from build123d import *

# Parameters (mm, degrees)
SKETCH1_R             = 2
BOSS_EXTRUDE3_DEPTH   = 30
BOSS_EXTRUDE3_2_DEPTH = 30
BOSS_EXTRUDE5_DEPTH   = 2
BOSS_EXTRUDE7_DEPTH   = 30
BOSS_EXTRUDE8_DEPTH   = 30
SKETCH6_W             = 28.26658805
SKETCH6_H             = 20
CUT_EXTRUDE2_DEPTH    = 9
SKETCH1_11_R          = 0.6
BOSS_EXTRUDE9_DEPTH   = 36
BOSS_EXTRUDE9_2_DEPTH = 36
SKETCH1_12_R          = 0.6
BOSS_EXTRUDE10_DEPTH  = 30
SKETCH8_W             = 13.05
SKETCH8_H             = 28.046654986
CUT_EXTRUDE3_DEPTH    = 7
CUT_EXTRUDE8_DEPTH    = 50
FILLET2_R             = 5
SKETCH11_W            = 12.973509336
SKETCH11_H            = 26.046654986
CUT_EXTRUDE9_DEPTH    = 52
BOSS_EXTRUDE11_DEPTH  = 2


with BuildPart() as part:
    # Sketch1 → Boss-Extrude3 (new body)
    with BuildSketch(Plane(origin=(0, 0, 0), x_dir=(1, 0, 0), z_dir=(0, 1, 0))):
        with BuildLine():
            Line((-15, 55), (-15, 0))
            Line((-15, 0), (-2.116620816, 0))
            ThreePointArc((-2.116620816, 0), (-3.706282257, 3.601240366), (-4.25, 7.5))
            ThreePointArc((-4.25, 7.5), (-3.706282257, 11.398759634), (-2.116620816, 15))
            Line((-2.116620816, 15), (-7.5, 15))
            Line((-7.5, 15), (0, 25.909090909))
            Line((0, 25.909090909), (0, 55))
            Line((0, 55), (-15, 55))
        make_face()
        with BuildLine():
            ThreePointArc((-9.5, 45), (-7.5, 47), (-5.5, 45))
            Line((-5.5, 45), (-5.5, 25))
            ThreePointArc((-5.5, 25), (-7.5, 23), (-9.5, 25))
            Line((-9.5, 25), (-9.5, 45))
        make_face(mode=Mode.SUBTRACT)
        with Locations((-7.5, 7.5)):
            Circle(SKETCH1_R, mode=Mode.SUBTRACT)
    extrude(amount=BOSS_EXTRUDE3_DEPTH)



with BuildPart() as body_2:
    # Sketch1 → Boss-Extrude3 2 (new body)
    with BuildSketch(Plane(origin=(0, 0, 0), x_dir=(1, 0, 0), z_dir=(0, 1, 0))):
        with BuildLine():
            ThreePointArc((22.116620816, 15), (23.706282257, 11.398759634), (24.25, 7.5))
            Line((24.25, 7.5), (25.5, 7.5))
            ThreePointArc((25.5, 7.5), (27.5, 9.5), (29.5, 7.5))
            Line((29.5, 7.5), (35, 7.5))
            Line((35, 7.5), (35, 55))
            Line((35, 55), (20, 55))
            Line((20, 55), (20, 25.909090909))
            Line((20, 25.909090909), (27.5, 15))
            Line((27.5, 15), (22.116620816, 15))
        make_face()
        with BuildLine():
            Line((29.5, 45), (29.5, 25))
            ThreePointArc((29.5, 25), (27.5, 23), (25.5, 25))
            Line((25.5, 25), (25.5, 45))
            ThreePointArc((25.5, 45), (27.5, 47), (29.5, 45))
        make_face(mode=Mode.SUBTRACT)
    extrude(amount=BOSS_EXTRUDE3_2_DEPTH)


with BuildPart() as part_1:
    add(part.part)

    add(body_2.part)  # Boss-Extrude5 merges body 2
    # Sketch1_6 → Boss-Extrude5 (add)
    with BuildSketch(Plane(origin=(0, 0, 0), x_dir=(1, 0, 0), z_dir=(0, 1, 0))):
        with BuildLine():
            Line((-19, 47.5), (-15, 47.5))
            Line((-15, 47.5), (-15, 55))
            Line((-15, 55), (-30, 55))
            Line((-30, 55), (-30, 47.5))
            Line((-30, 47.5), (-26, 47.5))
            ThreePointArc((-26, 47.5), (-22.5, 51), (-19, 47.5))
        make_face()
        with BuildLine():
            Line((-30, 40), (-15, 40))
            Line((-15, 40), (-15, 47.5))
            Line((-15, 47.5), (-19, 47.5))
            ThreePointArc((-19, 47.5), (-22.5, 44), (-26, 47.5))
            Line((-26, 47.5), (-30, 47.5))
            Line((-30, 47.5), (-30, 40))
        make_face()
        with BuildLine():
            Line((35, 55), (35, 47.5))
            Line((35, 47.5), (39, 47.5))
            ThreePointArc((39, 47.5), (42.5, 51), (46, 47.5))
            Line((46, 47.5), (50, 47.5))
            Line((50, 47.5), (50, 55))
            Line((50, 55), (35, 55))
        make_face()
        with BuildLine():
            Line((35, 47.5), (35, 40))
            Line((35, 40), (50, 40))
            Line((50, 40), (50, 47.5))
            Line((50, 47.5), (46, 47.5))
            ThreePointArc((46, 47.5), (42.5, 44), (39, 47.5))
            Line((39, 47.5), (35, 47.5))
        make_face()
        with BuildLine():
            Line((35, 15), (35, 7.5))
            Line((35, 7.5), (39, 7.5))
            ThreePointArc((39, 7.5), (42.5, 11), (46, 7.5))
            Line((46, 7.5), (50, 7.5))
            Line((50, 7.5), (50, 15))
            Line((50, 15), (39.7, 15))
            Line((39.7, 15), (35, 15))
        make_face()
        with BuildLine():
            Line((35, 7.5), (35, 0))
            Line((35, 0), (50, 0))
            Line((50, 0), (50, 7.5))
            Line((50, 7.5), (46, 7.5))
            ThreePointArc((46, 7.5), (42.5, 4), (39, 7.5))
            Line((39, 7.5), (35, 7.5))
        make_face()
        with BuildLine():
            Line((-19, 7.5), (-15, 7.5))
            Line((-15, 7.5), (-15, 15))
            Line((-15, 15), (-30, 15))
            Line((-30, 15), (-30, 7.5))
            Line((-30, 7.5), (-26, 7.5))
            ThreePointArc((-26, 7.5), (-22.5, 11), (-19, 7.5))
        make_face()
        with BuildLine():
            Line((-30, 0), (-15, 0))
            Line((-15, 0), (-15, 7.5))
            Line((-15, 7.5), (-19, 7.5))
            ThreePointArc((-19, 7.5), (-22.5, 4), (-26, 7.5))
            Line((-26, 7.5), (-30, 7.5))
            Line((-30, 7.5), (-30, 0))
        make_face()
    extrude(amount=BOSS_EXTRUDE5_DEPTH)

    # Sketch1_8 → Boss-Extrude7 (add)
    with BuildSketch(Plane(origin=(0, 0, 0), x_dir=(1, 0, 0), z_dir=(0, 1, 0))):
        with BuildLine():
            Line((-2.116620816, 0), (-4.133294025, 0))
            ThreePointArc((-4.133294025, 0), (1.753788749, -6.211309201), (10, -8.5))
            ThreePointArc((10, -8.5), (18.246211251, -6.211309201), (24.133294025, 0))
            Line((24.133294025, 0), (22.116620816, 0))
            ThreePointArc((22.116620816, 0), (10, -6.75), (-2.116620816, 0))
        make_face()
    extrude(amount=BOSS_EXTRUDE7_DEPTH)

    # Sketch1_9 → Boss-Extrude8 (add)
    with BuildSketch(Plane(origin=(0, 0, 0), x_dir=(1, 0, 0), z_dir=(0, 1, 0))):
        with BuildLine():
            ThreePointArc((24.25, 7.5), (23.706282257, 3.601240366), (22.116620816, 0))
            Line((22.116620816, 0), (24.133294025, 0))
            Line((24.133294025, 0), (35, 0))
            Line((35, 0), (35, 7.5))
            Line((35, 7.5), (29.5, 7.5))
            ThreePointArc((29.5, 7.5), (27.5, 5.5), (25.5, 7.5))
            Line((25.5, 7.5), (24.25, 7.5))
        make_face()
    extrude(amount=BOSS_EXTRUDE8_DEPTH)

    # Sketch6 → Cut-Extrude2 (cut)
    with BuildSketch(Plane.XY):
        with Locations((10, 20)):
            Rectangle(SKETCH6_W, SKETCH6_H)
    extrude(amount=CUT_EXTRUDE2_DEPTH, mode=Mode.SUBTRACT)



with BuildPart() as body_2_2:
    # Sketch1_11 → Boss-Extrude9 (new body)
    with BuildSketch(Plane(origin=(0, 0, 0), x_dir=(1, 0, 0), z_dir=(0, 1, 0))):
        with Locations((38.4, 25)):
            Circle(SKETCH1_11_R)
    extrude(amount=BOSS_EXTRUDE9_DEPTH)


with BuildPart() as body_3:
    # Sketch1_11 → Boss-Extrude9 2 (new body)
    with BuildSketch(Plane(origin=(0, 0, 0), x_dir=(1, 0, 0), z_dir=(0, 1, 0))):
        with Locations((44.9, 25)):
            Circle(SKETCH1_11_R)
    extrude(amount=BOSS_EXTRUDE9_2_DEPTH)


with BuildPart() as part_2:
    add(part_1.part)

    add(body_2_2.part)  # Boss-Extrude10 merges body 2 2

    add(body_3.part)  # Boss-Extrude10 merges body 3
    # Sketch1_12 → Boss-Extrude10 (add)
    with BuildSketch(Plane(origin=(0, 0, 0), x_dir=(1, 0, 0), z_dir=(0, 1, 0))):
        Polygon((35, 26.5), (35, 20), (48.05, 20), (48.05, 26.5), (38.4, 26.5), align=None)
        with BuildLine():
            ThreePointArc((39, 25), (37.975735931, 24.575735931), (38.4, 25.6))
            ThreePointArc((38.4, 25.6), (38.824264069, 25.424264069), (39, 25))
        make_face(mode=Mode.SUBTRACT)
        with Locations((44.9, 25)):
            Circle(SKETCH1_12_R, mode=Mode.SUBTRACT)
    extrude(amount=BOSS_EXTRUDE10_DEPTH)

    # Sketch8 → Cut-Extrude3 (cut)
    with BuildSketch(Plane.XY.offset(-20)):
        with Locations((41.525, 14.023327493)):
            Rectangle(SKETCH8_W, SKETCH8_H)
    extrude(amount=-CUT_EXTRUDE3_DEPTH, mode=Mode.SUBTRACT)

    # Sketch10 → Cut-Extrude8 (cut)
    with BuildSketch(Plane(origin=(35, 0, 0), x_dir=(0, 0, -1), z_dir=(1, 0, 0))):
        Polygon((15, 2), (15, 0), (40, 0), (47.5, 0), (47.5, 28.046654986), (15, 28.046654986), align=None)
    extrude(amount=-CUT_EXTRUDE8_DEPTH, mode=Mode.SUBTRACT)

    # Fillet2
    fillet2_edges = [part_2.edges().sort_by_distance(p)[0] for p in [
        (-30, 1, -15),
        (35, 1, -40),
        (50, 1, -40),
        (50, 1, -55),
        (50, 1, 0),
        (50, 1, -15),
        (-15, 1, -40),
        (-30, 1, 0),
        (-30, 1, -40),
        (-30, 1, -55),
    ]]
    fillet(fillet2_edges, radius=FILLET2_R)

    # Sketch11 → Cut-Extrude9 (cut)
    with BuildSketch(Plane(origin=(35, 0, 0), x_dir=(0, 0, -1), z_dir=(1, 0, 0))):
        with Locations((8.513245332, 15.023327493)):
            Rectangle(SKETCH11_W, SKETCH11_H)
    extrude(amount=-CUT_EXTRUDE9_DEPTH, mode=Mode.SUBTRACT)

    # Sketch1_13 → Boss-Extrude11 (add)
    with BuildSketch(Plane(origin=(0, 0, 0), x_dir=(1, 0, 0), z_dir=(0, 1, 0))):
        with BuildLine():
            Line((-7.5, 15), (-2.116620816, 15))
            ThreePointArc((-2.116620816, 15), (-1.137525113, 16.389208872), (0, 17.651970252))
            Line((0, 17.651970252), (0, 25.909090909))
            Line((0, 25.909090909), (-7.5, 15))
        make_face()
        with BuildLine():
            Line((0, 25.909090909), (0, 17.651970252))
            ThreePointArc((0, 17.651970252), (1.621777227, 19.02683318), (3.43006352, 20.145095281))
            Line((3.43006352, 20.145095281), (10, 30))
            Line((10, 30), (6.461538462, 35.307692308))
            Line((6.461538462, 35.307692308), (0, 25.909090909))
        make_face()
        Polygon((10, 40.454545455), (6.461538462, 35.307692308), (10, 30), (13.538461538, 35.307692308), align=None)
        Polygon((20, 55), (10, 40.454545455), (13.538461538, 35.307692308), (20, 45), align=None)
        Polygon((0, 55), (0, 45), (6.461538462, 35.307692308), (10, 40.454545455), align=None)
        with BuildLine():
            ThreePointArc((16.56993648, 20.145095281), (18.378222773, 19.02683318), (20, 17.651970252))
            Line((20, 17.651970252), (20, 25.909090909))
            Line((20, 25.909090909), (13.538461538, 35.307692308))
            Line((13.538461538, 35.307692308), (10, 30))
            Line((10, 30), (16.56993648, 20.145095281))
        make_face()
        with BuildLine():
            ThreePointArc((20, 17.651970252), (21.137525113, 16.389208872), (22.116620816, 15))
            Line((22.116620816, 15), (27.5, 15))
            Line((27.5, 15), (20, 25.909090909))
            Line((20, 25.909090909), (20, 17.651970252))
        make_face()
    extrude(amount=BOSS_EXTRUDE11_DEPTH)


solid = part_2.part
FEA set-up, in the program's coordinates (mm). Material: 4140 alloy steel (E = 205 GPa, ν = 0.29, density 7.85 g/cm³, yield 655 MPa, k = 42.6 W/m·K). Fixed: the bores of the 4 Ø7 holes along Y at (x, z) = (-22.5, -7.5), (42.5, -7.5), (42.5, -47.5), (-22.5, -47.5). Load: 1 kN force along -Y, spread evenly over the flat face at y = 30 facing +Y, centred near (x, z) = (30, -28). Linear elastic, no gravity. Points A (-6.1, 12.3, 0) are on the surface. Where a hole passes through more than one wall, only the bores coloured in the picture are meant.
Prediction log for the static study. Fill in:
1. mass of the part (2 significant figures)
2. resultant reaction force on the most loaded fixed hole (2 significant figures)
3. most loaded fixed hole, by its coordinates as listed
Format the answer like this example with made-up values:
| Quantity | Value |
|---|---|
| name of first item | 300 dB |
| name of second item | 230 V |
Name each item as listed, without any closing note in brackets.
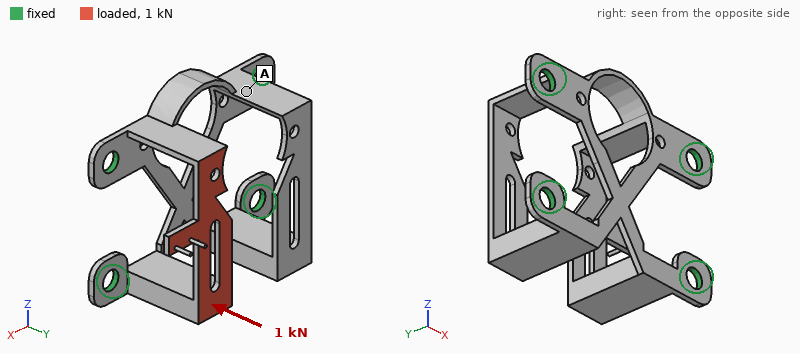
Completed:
| Quantity | Value |
|---|---|
| mass of the part | 110 g |
| resultant reaction force on the most loaded fixed hole | 580 N |
| most loaded fixed hole, by its coordinates as listed | (42.5, -47.5) |
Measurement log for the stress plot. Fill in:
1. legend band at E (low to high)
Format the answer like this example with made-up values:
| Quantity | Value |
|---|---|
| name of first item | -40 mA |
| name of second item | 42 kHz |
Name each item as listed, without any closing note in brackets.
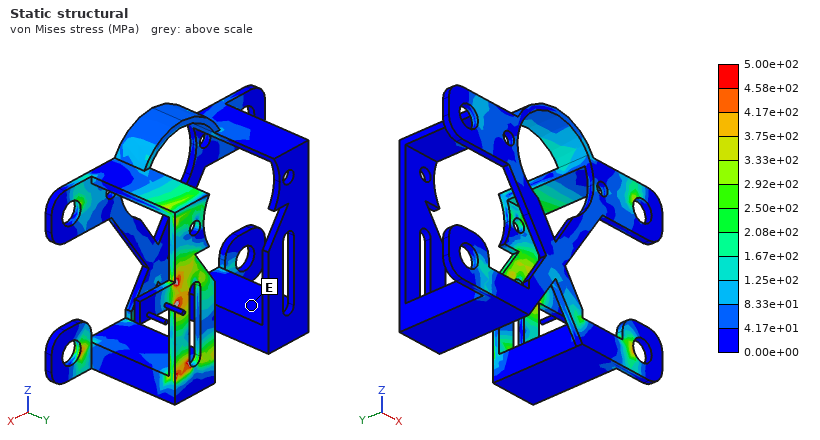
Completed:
| Quantity | Value |
|---|---|
| legend band at E | 0.00e+00 to 4.17e+01 MPa |
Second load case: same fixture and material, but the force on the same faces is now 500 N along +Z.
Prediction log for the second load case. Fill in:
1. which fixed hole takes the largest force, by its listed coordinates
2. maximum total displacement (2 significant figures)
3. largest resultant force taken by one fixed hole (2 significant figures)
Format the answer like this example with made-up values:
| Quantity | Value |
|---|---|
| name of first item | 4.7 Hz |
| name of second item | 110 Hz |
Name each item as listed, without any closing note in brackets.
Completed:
| Quantity | Value |
|---|---|
| which fixed hole takes the largest force, by its listed coordinates | (42.5, -47.5) |
| maximum total displacement | 0.43 mm |
| largest resultant force taken by one fixed hole | 360 N |
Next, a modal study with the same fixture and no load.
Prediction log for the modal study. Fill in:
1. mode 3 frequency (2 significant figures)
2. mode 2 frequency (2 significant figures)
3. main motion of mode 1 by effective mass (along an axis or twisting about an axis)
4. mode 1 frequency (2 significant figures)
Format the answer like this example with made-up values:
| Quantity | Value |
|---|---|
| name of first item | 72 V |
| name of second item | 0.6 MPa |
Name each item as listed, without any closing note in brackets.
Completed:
| Quantity | Value |
|---|---|
| mode 3 frequency | 1200 Hz |
| mode 2 frequency | 1200 Hz |
| main motion of mode 1 by effective mass | along Y |
| mode 1 frequency | 940 Hz |
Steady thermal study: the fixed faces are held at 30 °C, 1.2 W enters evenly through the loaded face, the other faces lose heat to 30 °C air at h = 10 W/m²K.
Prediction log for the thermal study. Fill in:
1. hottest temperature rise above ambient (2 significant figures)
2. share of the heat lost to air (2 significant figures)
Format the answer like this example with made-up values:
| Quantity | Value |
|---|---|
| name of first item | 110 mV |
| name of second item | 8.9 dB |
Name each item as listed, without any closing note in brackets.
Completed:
| Quantity | Value |
|---|---|
| hottest temperature rise above ambient | 18 K |
| share of the heat lost to air | 30 % |
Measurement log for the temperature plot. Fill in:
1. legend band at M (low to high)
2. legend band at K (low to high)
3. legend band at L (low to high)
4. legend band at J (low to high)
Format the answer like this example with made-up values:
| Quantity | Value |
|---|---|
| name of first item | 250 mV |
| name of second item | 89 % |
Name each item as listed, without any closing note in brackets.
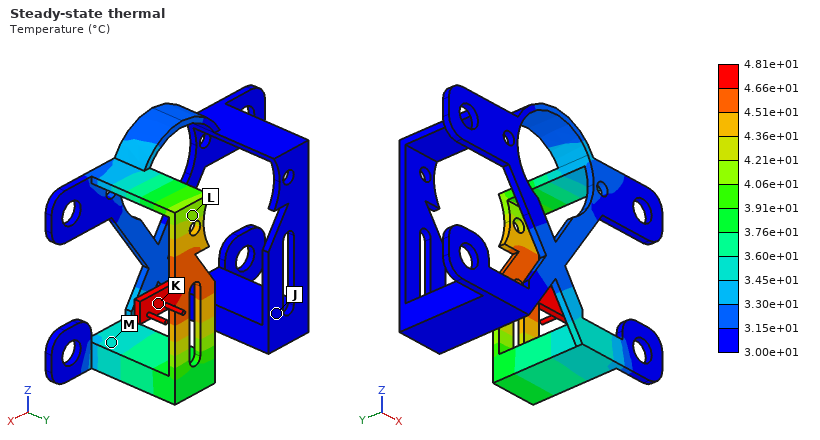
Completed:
| Quantity | Value |
|---|---|
| legend band at M | 3.45e+01 to 3.60e+01 °C |
| legend band at K | 4.66e+01 to 4.81e+01 °C |
| legend band at L | 4.06e+01 to 4.21e+01 °C |
| legend band at J | 3.00e+01 to 3.15e+01 °C |
